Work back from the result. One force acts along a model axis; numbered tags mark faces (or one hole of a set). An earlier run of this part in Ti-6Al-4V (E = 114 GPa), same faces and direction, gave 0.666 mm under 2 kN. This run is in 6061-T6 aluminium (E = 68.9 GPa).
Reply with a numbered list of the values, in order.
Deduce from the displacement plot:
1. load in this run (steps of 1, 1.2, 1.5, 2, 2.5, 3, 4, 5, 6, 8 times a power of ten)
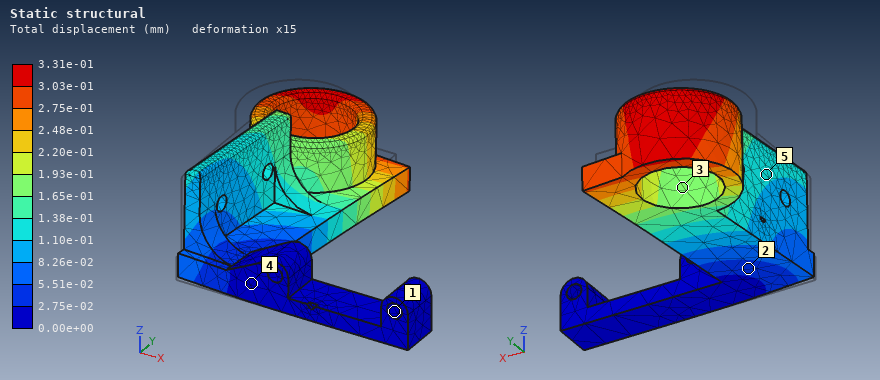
1. 600 N
